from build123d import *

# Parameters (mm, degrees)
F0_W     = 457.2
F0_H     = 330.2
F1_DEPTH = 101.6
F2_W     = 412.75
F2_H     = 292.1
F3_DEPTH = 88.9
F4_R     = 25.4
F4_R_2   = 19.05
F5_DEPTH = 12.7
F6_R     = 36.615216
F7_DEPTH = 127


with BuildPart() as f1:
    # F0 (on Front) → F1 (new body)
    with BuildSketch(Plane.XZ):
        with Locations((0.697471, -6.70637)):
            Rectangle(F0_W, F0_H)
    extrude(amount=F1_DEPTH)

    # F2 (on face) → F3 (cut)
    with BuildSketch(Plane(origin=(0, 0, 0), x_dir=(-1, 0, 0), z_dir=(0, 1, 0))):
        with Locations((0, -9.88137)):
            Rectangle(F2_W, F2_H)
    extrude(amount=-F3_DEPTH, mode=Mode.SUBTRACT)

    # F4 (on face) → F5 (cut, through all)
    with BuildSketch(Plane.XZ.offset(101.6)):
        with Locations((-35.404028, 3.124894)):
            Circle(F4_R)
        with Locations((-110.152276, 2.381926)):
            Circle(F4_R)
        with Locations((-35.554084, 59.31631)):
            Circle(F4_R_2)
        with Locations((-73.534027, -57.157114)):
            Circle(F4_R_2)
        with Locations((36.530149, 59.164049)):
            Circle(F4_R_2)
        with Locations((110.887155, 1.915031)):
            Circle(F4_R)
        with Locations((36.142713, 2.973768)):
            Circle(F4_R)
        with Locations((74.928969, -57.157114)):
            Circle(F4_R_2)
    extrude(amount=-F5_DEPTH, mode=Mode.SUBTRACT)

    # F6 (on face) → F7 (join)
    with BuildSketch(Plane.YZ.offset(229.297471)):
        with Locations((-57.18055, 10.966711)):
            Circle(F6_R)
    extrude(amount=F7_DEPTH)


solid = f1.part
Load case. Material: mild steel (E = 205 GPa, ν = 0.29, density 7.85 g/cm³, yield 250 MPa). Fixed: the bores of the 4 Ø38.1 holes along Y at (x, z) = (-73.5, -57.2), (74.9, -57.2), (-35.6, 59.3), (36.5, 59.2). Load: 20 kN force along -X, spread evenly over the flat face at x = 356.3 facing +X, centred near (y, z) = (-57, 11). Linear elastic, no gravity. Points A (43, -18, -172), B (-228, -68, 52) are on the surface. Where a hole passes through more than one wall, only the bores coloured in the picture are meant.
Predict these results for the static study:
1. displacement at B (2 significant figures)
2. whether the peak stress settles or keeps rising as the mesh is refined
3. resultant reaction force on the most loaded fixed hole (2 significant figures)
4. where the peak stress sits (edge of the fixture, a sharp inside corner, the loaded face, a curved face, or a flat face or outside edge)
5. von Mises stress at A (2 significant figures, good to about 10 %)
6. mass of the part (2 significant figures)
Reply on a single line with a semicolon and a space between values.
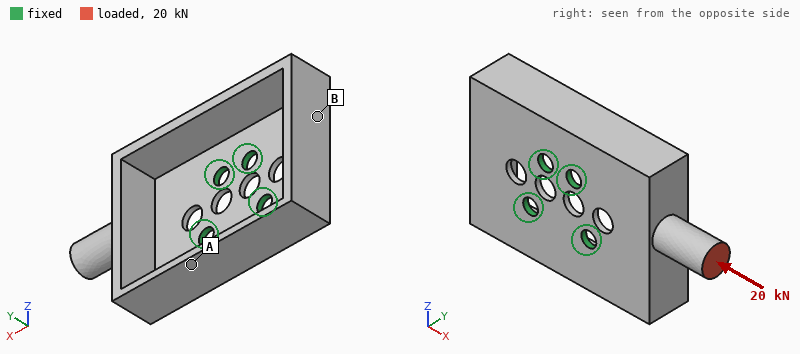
0.089 mm; keeps rising; 9.0 kN; edge of the fixture; 7.2 MPa; 39 kg
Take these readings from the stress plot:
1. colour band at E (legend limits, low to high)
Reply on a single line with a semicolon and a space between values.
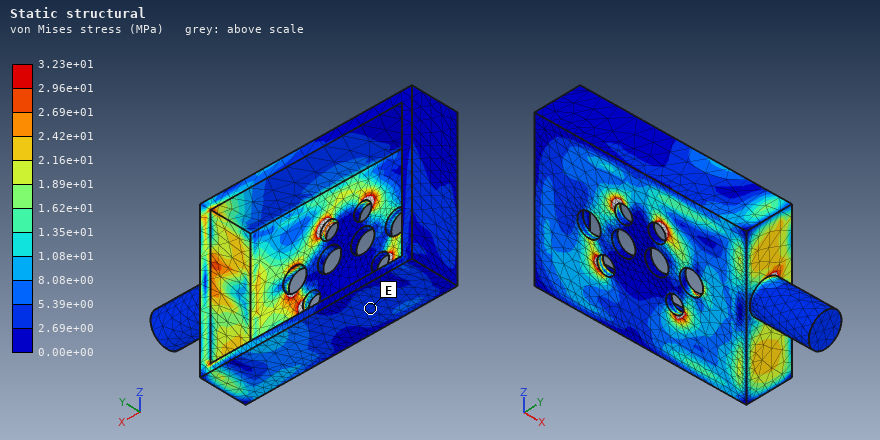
2.69e+00 to 5.39e+00 MPa
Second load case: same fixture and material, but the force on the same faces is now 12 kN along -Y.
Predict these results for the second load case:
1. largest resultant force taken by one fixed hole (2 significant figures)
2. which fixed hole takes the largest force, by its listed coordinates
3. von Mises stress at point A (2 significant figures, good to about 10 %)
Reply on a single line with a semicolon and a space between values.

18 kN; (36.5, 59.2); 33 MPa
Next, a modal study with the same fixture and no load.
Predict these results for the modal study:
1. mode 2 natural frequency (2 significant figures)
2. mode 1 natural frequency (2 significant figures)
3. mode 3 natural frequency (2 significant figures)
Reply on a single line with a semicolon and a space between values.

350 Hz; 210 Hz; 360 Hz
